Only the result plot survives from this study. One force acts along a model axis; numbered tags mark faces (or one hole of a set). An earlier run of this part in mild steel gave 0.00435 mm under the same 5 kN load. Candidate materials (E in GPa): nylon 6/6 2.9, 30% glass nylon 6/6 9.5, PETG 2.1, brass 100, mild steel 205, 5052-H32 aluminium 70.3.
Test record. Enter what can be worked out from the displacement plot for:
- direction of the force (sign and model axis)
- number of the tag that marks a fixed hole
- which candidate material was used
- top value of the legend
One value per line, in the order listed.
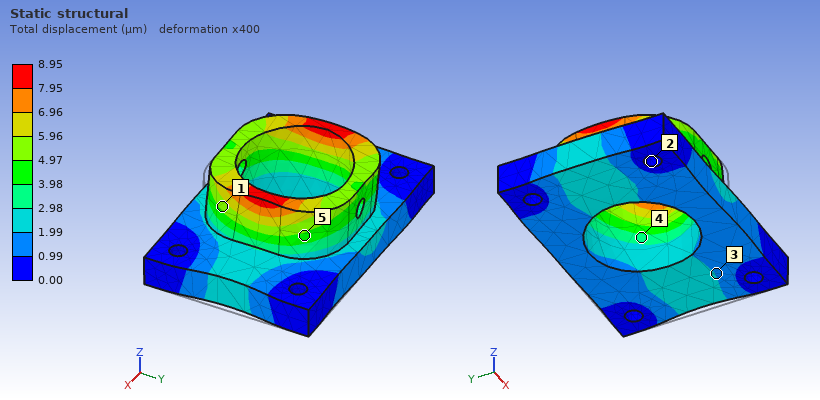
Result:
-X
2
brass
8.95 µm
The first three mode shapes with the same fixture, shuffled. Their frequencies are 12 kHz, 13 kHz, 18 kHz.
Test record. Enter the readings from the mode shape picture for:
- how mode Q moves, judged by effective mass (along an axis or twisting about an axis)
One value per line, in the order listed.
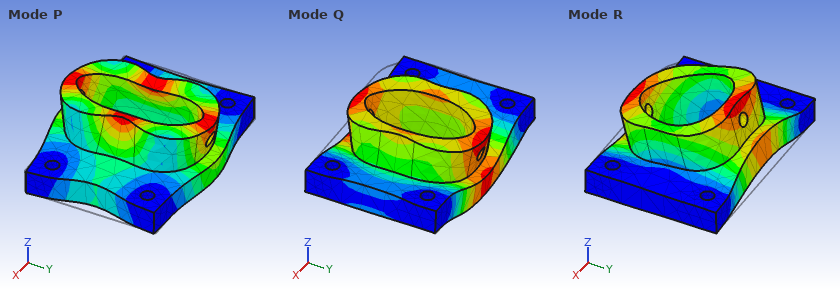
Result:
along Z
